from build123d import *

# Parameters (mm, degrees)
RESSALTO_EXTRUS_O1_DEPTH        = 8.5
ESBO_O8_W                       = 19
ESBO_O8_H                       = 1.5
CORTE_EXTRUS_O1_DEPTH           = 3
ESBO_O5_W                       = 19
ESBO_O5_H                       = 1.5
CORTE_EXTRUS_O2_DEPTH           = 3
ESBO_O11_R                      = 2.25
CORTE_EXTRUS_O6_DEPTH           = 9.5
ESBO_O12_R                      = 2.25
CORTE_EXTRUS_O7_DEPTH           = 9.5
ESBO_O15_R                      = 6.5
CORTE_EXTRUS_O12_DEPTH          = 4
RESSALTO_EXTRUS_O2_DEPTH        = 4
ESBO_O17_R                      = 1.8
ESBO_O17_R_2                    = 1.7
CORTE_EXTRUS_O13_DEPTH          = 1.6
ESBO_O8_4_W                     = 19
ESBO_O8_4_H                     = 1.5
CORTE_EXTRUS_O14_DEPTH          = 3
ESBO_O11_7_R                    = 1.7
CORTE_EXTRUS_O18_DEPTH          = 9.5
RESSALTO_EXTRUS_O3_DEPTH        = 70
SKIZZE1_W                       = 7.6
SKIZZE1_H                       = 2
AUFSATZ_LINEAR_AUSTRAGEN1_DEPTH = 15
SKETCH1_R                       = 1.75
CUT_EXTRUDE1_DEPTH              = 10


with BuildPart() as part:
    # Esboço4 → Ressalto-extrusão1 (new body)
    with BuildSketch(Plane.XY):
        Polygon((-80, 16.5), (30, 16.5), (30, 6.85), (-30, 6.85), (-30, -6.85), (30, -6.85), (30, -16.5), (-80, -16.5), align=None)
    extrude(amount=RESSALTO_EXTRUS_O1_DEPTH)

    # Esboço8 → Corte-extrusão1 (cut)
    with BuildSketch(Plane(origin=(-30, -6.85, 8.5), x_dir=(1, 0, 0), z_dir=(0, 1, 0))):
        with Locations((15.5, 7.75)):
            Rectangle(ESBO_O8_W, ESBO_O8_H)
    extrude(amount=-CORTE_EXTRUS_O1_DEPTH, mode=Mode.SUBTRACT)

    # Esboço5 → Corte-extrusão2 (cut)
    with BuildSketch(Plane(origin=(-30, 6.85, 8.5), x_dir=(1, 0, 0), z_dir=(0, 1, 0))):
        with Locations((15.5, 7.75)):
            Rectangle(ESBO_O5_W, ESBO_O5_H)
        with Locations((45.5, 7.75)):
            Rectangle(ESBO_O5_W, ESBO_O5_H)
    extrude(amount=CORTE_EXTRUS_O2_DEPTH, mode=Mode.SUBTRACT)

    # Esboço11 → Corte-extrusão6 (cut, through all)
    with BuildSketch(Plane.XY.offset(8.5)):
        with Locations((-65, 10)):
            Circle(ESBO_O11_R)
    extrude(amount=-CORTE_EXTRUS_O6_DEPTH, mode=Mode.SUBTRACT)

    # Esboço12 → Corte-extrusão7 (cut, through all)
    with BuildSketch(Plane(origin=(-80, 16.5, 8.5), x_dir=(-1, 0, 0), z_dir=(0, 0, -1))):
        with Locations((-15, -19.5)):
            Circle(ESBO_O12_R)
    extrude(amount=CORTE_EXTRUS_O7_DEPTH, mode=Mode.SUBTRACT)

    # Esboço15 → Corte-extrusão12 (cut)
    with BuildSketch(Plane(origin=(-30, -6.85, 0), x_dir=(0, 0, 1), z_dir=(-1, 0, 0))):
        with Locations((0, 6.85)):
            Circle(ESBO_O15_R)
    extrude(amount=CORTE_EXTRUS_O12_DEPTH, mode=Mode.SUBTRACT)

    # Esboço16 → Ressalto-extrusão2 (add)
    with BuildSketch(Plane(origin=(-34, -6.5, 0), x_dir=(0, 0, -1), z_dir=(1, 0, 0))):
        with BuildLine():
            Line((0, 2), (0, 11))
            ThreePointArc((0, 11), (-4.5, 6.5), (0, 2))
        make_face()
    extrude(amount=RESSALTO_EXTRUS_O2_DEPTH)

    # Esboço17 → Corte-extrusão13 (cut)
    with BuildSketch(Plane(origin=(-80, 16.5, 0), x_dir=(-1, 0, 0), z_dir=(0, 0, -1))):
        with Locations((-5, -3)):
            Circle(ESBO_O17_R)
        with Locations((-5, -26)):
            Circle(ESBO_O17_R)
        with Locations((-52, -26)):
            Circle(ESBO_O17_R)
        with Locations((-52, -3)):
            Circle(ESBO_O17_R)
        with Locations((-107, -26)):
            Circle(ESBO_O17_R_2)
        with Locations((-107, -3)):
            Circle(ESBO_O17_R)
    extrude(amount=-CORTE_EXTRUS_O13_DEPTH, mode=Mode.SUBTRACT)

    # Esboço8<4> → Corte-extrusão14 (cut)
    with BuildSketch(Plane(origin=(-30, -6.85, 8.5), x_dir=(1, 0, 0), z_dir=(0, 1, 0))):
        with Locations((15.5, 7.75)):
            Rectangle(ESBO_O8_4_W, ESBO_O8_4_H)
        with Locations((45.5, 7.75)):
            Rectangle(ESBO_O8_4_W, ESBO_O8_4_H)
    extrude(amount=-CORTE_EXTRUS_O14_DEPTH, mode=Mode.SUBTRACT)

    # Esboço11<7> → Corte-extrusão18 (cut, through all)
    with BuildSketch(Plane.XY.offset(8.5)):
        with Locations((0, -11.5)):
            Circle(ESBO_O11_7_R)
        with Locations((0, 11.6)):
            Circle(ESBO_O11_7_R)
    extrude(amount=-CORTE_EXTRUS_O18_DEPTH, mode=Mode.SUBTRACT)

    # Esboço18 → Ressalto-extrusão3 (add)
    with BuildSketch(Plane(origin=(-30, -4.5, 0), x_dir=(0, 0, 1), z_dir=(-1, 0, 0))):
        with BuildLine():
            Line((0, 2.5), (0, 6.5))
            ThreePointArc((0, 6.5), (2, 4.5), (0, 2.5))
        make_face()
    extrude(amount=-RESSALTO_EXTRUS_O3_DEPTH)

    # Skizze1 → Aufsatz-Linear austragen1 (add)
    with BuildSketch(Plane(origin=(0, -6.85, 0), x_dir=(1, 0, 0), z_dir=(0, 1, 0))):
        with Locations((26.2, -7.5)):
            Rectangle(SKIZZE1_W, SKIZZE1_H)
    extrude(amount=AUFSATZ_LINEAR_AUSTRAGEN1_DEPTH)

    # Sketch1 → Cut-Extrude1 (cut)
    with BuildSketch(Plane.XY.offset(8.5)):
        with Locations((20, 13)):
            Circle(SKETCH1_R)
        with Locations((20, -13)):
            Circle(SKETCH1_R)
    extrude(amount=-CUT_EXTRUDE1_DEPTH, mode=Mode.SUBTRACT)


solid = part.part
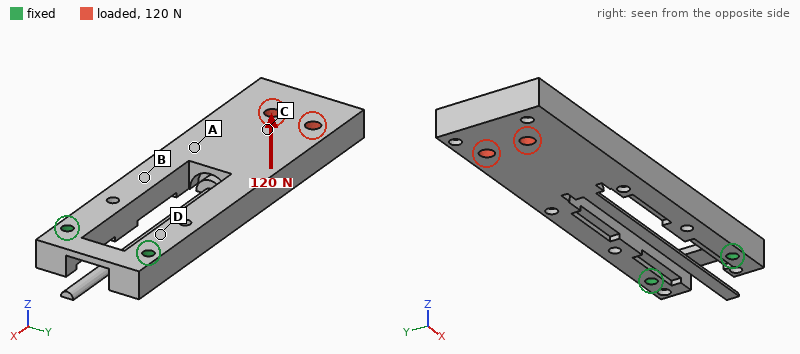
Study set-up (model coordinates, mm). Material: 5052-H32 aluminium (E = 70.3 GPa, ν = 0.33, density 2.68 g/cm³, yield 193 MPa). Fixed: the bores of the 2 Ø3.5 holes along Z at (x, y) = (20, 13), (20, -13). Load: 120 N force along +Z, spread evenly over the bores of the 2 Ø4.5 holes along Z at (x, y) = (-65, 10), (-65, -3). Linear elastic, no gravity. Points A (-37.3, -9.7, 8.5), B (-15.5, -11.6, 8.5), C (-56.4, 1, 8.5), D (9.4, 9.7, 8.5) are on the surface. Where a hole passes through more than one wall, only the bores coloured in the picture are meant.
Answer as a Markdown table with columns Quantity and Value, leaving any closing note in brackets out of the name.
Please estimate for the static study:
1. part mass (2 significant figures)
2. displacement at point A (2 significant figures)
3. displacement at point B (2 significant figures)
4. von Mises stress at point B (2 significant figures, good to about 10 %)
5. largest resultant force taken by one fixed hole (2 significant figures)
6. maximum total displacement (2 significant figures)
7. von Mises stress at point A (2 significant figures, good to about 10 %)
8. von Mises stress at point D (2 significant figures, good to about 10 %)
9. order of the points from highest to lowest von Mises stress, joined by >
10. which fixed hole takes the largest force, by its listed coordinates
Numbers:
| Quantity | Value |
|---|---|
| part mass | 63 g |
| displacement at point A | 0.22 mm |
| displacement at point B | 0.092 mm |
| von Mises stress at point B | 28 MPa |
| largest resultant force taken by one fixed hole | 67 N |
| maximum total displacement | 0.51 mm |
| von Mises stress at point A | 12 MPa |
| von Mises stress at point D | 42 MPa |
| order of the points from highest to lowest von Mises stress, joined by > | D > B > A > C |
| which fixed hole takes the largest force, by its listed coordinates | (20, 13) |
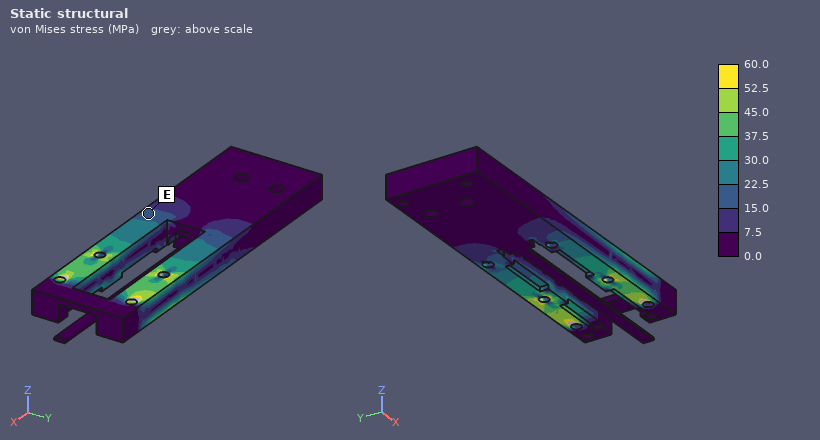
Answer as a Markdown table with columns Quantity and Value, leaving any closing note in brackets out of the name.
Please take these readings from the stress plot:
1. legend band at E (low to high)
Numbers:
| Quantity | Value |
|---|---|
| legend band at E | 15.0 to 22.5 MPa |
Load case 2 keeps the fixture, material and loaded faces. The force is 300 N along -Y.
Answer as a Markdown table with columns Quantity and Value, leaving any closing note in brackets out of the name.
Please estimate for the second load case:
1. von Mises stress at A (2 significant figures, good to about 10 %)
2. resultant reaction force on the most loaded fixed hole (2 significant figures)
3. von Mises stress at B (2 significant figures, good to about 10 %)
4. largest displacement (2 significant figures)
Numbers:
| Quantity | Value |
|---|---|
| von Mises stress at A | 9.0 MPa |
| resultant reaction force on the most loaded fixed hole | 760 N |
| von Mises stress at B | 9.7 MPa |
| largest displacement | 0.11 mm |
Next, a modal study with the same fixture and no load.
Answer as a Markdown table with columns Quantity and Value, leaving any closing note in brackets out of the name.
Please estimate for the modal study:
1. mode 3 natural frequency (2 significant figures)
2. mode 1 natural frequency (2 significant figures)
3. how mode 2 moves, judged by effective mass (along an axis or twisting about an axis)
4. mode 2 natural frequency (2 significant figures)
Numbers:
| Quantity | Value |
|---|---|
| mode 3 natural frequency | 560 Hz |
| mode 1 natural frequency | 300 Hz |
| how mode 2 moves, judged by effective mass | along Z |
| mode 2 natural frequency | 520 Hz |
